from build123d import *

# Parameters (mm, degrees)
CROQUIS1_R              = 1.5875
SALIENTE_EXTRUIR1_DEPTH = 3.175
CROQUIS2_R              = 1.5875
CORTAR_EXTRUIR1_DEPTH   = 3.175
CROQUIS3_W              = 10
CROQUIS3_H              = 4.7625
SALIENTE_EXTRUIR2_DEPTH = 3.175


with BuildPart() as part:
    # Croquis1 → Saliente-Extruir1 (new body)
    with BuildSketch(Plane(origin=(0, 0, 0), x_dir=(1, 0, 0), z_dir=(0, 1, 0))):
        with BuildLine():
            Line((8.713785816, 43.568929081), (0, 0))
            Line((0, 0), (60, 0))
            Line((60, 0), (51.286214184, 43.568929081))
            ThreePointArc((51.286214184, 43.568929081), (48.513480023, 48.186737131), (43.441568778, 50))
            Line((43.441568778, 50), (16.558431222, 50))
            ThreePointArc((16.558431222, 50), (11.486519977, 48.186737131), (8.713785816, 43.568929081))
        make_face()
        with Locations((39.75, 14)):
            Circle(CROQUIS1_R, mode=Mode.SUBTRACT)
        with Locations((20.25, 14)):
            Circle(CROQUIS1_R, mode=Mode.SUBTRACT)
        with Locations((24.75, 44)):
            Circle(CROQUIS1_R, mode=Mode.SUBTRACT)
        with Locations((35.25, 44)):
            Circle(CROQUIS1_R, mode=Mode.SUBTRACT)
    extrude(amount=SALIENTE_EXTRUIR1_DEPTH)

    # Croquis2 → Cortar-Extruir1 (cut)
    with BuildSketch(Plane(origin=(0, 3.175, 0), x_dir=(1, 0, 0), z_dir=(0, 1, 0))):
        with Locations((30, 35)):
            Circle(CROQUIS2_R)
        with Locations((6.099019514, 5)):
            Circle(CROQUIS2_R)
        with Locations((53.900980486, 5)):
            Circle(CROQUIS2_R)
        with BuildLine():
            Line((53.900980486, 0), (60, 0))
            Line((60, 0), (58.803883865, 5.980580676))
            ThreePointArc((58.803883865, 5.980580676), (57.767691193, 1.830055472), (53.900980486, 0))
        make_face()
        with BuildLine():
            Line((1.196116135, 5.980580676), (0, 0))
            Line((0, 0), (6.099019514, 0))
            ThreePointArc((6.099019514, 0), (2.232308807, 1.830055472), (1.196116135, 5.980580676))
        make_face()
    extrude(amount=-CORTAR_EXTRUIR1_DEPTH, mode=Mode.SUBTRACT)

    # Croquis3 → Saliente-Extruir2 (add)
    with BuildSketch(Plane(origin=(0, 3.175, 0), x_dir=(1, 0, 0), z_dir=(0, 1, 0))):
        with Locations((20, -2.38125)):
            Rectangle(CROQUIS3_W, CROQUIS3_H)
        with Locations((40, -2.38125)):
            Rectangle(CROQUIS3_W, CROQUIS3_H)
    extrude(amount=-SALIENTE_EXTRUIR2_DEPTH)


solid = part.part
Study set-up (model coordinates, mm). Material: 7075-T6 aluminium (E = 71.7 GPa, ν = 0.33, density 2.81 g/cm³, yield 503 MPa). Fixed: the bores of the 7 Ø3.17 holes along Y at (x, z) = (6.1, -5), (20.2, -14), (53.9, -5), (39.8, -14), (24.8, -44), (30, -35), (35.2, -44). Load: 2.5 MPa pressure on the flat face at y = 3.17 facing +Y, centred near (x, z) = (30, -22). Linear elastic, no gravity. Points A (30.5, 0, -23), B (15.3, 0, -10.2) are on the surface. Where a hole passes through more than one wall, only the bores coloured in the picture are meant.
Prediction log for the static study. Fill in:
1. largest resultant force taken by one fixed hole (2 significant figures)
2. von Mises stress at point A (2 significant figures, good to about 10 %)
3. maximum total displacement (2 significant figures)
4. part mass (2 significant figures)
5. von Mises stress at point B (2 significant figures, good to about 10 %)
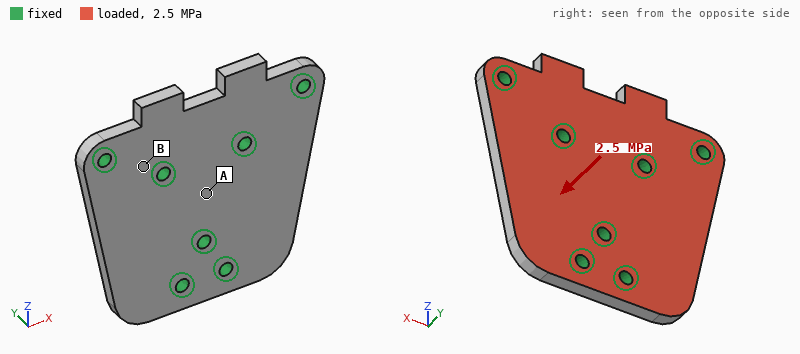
1.3 kN
32 MPa
0.13 mm
22 g
94 MPa
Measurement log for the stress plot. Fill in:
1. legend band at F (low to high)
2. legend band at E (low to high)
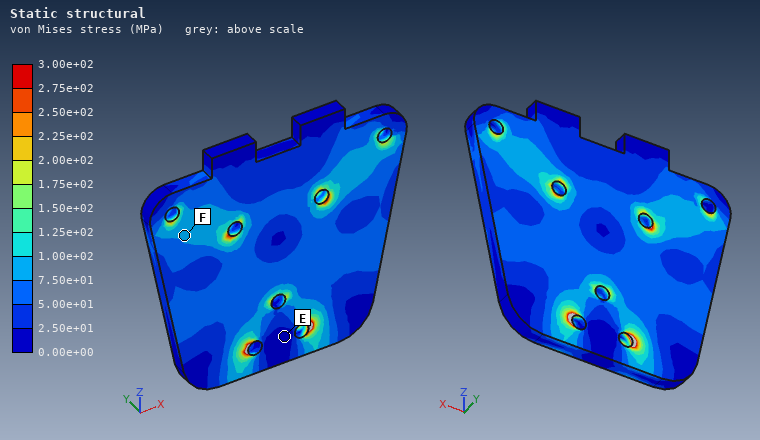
7.50e+01 to 1.00e+02 MPa
0.00e+00 to 2.50e+01 MPa
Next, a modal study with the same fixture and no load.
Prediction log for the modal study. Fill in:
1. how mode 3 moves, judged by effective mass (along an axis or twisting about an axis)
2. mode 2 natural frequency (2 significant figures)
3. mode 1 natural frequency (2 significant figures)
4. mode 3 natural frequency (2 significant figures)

along Y
9600 Hz
9600 Hz
12 kHz
